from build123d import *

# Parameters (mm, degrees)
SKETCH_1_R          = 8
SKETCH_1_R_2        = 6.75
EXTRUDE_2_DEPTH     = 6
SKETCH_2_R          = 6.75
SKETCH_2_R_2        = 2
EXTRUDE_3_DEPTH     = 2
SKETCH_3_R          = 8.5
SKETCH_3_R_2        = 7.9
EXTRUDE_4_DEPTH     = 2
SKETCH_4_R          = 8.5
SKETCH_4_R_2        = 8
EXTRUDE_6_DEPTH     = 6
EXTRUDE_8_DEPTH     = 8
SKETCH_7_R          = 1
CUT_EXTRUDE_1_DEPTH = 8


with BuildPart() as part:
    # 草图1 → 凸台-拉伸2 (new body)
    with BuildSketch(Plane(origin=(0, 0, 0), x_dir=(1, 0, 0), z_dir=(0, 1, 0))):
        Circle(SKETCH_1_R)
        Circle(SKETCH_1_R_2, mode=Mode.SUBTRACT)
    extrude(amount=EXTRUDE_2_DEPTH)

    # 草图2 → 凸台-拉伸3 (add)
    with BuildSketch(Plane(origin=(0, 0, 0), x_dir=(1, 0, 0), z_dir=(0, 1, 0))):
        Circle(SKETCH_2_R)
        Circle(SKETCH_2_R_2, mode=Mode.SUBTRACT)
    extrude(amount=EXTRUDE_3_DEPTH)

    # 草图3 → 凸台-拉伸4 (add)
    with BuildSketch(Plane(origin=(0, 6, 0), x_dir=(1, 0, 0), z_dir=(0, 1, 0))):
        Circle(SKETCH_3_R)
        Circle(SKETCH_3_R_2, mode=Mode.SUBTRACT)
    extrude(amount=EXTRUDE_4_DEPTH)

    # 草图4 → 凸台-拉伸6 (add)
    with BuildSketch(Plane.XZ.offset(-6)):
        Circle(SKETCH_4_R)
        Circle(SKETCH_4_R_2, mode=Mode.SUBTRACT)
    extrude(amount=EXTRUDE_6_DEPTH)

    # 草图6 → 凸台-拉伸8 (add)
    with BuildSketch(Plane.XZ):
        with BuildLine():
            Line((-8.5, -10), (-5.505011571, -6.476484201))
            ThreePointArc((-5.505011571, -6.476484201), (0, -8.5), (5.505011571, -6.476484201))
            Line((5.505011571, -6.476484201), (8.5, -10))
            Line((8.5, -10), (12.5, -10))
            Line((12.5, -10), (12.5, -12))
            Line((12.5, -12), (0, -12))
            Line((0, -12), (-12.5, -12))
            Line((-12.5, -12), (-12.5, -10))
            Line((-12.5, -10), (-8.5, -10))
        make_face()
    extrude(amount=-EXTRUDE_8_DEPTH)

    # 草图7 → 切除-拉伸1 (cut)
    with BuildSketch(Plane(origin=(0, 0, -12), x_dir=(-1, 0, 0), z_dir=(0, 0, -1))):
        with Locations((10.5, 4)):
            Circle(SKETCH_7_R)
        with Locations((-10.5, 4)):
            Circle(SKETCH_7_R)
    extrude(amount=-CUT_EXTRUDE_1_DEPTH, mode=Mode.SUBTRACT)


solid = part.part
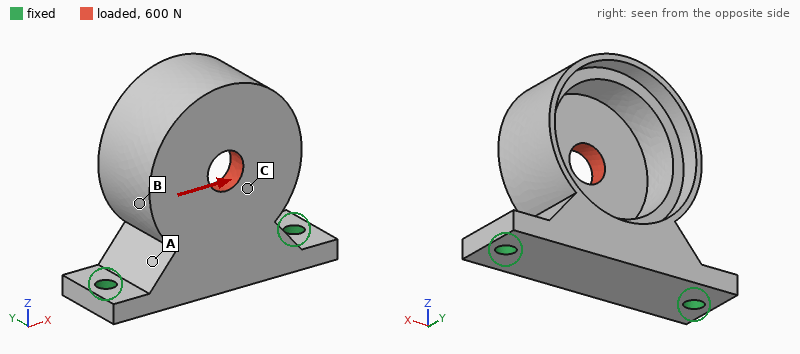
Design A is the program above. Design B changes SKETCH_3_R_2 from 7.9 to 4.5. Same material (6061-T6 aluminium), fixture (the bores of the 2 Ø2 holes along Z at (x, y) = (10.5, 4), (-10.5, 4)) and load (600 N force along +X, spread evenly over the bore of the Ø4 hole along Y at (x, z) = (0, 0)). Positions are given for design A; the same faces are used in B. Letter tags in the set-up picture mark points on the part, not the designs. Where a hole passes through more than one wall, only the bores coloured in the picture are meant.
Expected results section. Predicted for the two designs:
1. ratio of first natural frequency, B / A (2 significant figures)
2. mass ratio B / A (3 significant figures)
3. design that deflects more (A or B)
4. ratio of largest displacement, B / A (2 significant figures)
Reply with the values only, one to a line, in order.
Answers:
0.92
1.18
A
0.69
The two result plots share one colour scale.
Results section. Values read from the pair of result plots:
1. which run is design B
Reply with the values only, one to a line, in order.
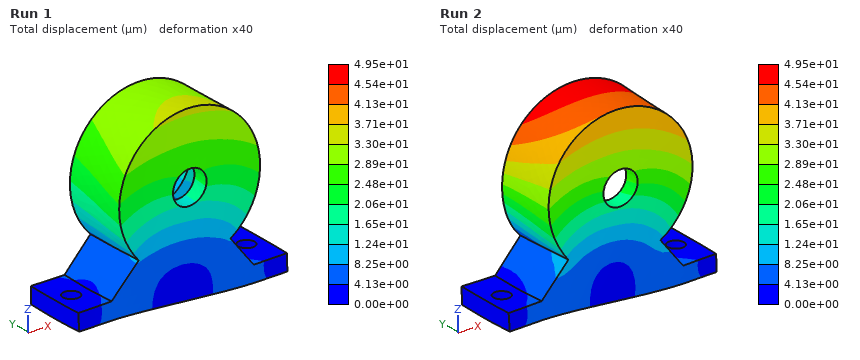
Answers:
Run 1
